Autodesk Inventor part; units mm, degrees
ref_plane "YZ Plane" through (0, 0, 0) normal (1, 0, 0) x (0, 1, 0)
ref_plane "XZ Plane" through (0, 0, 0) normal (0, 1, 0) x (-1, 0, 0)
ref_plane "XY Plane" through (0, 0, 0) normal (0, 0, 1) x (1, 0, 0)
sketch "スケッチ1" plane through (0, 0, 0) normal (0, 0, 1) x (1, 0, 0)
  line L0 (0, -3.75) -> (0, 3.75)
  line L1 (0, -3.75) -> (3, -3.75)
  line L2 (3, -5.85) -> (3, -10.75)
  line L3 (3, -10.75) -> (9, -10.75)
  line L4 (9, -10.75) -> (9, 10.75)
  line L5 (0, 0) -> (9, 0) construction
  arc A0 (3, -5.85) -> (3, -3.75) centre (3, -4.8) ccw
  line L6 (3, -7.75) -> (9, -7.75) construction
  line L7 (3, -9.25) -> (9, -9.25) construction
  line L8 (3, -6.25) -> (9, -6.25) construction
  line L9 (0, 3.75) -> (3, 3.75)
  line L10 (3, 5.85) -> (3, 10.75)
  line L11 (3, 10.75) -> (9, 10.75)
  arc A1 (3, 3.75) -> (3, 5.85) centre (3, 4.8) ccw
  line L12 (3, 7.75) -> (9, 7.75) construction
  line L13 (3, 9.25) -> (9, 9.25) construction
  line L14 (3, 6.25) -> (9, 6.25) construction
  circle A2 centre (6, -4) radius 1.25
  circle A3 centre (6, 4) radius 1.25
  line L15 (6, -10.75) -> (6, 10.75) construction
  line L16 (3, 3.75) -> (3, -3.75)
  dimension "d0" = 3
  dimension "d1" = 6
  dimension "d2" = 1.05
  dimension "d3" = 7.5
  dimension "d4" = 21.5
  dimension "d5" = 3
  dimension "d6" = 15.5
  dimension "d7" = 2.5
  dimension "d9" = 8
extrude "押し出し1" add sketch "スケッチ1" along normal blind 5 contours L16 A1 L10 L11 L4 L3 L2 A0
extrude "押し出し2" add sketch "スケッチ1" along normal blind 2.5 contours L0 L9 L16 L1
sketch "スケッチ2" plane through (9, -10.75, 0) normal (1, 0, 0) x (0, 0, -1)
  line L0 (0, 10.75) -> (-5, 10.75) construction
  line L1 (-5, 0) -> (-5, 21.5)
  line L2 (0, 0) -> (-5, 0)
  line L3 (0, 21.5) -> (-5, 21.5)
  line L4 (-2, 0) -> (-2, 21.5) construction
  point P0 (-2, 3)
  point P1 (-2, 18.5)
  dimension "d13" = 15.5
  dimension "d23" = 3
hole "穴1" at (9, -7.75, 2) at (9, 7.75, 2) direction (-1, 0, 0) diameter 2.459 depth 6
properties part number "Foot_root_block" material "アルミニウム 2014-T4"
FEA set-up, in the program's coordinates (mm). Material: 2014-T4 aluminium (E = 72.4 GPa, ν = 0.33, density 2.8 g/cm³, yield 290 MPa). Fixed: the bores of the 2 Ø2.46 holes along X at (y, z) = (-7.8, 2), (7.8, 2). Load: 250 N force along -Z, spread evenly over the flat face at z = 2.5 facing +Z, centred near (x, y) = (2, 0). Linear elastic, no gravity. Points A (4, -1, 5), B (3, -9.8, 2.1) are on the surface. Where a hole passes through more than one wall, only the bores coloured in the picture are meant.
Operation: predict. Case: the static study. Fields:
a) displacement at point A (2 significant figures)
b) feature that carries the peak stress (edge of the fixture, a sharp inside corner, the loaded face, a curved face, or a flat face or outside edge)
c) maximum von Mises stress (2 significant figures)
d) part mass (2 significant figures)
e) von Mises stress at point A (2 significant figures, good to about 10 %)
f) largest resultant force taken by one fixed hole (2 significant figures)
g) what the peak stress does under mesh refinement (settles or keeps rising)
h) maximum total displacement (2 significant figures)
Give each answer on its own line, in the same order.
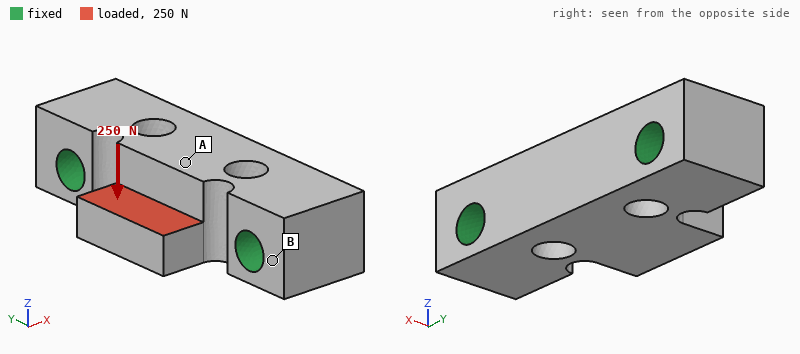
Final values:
7.9 µm
a curved face
160 MPa
1.6 g
27 MPa
130 N
settles
20 µm
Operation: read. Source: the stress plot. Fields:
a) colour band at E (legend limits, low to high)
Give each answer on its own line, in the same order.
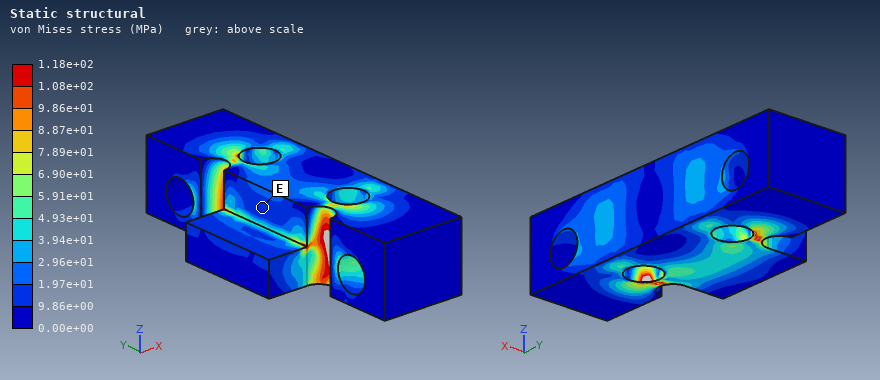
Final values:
9.86e+00 to 1.97e+01 MPa
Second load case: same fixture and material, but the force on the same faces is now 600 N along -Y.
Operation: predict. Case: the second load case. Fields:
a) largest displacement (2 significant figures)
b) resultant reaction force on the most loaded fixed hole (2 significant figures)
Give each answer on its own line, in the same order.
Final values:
15 µm
360 N
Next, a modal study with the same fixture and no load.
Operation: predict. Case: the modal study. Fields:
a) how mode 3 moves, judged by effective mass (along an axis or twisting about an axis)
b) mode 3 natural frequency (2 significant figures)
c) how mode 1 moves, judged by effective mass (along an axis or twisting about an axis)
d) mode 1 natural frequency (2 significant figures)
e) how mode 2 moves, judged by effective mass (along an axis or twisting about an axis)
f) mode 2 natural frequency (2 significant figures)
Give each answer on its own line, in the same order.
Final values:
along Z
73 kHz
along Z
42 kHz
along X
59 kHz
